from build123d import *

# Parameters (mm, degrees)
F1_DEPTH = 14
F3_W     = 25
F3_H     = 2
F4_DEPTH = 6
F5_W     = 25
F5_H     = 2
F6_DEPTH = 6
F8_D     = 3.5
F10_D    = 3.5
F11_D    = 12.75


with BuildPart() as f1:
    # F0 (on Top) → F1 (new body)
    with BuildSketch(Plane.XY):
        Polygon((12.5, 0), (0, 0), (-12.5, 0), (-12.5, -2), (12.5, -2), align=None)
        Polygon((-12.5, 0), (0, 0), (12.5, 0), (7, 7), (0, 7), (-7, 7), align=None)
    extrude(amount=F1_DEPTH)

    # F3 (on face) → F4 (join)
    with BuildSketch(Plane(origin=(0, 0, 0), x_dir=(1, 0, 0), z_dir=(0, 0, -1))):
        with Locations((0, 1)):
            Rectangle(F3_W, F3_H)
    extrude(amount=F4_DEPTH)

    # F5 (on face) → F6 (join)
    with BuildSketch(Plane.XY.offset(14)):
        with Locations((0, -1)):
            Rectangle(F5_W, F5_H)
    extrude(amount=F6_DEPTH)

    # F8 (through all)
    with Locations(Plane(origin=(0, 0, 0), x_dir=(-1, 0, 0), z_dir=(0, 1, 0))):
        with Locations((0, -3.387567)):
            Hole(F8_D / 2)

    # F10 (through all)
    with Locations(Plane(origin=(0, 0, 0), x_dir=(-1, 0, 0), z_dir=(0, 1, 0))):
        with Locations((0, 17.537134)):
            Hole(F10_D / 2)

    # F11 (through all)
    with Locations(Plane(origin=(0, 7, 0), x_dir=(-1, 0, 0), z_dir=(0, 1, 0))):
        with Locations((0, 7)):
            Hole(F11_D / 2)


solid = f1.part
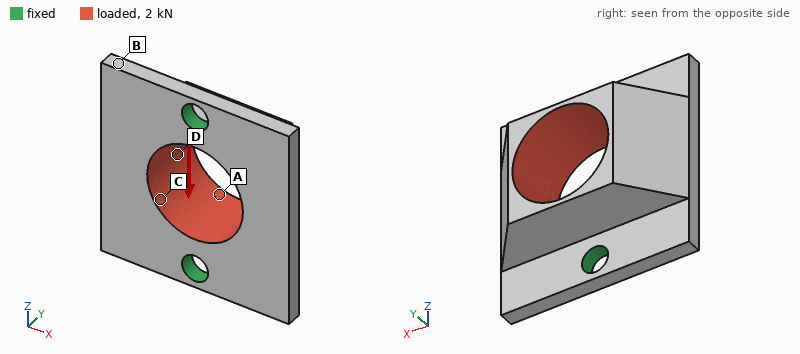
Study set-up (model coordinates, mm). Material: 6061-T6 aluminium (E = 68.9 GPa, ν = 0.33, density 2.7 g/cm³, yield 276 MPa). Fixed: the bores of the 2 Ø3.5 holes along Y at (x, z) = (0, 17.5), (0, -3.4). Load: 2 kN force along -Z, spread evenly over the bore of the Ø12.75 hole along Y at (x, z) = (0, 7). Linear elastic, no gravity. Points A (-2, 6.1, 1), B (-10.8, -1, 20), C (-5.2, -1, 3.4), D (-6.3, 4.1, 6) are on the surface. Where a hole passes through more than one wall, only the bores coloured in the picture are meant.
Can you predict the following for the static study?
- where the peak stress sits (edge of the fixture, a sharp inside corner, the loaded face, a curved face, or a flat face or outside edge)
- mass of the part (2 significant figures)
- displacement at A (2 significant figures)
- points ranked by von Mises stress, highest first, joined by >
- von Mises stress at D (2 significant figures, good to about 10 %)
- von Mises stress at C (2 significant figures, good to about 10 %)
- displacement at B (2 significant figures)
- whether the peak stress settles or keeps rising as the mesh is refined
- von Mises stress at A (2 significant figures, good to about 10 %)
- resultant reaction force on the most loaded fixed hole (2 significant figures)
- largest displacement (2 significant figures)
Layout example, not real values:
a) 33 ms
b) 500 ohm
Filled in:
a) edge of the fixture
b) 5.5 g
c) 23 µm
d) A > C > D > B
e) 27 MPa
f) 49 MPa
g) 13 µm
h) keeps rising
i) 67 MPa
j) 1.1 kN
k) 28 µm
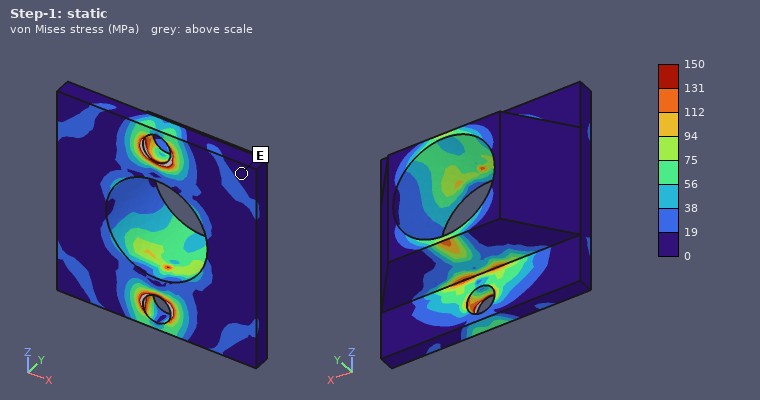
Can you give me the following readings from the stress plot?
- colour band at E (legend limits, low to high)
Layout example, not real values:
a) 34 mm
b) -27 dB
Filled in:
a) 0 to 19 MPa
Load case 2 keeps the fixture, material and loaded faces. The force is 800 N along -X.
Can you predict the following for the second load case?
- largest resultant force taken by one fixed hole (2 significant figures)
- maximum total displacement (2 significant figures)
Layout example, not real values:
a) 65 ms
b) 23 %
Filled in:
a) 400 N
b) 46 µm
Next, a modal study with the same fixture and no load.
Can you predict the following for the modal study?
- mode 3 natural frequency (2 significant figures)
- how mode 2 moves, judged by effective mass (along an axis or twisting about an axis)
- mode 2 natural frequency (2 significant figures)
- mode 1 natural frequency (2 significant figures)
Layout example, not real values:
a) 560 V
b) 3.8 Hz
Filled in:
a) 22 kHz
b) along Y
c) 17 kHz
d) 7600 Hz
